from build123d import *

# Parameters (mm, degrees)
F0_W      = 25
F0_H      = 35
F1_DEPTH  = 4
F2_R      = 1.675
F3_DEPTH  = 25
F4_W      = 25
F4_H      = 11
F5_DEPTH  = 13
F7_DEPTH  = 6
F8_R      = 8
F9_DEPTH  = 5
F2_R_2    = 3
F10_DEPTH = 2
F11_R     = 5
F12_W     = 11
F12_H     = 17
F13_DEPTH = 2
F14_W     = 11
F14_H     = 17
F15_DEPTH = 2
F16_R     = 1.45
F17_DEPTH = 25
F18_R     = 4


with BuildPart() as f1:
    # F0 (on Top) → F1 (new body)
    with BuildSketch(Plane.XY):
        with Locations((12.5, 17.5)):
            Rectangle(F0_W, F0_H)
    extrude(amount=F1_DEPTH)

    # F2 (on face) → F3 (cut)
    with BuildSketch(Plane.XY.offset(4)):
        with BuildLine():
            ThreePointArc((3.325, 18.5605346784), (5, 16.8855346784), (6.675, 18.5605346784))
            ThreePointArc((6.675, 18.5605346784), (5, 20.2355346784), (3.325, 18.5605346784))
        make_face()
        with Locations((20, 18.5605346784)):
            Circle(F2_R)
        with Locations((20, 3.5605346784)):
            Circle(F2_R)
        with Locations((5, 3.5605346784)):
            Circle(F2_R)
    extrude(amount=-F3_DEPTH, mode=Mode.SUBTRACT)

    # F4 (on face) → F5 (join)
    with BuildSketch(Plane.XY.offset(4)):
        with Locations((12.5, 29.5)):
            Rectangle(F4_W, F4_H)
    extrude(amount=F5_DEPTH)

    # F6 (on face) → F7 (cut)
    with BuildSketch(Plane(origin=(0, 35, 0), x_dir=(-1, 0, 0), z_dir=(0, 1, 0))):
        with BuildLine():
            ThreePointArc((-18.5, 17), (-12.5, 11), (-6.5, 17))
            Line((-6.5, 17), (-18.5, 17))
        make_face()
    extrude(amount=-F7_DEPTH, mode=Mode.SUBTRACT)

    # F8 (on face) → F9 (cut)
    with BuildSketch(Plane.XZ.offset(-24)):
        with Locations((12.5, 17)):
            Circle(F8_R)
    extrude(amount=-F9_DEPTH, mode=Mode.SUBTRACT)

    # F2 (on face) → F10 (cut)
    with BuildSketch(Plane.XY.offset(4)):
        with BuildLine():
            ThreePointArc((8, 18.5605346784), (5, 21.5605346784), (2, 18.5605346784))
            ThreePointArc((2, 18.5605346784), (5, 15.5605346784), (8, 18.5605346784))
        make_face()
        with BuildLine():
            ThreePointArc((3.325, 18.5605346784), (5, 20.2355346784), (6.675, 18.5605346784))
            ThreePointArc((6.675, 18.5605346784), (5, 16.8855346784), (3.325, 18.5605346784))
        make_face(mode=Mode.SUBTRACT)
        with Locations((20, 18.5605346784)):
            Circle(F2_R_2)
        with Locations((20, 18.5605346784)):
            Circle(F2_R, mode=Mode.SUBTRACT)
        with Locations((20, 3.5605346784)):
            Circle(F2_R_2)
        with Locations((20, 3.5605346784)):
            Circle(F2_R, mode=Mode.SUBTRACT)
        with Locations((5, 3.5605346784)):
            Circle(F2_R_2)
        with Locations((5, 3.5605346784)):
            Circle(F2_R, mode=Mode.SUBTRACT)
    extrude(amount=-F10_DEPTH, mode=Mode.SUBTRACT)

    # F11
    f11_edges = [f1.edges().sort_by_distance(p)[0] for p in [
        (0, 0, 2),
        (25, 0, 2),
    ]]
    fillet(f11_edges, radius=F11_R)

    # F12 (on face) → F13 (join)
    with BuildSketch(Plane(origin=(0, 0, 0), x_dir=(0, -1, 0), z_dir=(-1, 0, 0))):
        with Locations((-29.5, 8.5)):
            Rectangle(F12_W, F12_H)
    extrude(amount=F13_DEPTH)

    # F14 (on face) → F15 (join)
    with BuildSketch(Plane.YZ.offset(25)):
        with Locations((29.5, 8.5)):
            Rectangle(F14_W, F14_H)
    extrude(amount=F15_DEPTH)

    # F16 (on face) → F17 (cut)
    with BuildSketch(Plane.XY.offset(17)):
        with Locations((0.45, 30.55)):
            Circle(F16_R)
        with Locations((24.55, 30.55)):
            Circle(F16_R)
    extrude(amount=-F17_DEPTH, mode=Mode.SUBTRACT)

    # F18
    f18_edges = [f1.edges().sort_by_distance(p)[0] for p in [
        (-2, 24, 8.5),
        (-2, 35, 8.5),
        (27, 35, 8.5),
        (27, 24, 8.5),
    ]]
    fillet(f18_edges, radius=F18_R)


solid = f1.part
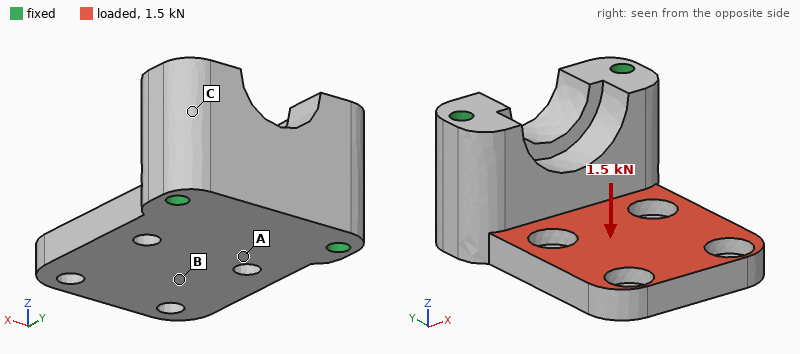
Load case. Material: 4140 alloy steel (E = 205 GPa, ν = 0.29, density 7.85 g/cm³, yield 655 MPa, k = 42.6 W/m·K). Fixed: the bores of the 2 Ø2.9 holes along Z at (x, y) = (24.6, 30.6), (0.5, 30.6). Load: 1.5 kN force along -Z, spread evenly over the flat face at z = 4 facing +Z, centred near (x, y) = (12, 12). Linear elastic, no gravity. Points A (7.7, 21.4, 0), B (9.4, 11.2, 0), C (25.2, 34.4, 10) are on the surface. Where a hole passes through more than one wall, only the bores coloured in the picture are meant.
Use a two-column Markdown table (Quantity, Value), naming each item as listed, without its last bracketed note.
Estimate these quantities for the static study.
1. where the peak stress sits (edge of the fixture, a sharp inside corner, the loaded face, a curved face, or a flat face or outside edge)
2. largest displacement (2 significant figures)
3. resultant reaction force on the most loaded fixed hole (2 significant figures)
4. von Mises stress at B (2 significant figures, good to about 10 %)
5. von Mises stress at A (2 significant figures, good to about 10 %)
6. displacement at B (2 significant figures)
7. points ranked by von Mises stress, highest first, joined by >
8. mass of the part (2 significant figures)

| Quantity | Value |
|---|---|
| where the peak stress sits | the loaded face |
| largest displacement | 0.16 mm |
| resultant reaction force on the most loaded fixed hole | 760 N |
| von Mises stress at B | 50 MPa |
| von Mises stress at A | 240 MPa |
| displacement at B | 0.074 mm |
| points ranked by von Mises stress, highest first, joined by > | A > B > C |
| mass of the part | 49 g |
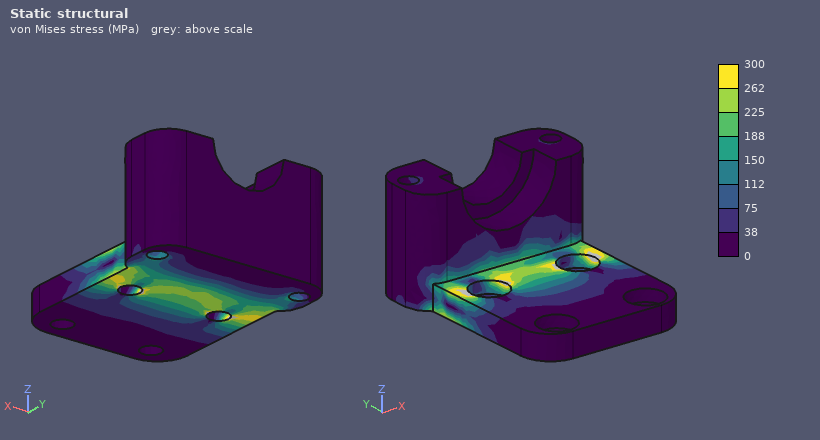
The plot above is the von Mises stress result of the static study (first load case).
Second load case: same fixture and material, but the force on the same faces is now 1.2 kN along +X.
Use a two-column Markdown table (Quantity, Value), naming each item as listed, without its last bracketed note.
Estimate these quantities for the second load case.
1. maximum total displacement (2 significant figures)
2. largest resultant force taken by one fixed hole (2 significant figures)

| Quantity | Value |
|---|---|
| maximum total displacement | 14 µm |
| largest resultant force taken by one fixed hole | 1.1 kN |
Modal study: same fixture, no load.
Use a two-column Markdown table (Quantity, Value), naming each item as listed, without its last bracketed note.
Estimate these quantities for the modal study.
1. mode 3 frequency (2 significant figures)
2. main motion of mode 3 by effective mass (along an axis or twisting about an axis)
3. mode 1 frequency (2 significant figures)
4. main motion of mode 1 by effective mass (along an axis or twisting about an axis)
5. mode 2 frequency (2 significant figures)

| Quantity | Value |
|---|---|
| mode 3 frequency | 18 kHz |
| main motion of mode 3 by effective mass | along X |
| mode 1 frequency | 4800 Hz |
| main motion of mode 1 by effective mass | along Z |
| mode 2 frequency | 12 kHz |
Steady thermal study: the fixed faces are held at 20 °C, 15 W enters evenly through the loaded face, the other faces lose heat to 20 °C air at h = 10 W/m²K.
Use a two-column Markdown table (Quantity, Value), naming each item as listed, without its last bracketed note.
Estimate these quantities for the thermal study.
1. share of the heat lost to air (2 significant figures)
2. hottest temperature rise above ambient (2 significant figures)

| Quantity | Value |
|---|---|
| share of the heat lost to air | 4.2 % |
| hottest temperature rise above ambient | 65 K |
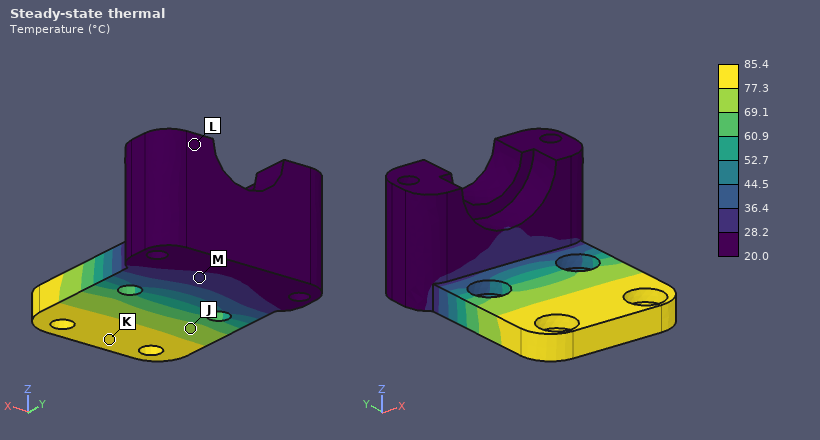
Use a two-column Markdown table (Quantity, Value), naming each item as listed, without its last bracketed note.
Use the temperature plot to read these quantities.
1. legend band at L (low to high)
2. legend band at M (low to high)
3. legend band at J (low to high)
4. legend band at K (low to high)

| Quantity | Value |
|---|---|
| legend band at L | 20.0 to 28.2 °C |
| legend band at M | 28.2 to 36.4 °C |
| legend band at J | 69.1 to 77.3 °C |
| legend band at K | 77.3 to 85.4 °C |
